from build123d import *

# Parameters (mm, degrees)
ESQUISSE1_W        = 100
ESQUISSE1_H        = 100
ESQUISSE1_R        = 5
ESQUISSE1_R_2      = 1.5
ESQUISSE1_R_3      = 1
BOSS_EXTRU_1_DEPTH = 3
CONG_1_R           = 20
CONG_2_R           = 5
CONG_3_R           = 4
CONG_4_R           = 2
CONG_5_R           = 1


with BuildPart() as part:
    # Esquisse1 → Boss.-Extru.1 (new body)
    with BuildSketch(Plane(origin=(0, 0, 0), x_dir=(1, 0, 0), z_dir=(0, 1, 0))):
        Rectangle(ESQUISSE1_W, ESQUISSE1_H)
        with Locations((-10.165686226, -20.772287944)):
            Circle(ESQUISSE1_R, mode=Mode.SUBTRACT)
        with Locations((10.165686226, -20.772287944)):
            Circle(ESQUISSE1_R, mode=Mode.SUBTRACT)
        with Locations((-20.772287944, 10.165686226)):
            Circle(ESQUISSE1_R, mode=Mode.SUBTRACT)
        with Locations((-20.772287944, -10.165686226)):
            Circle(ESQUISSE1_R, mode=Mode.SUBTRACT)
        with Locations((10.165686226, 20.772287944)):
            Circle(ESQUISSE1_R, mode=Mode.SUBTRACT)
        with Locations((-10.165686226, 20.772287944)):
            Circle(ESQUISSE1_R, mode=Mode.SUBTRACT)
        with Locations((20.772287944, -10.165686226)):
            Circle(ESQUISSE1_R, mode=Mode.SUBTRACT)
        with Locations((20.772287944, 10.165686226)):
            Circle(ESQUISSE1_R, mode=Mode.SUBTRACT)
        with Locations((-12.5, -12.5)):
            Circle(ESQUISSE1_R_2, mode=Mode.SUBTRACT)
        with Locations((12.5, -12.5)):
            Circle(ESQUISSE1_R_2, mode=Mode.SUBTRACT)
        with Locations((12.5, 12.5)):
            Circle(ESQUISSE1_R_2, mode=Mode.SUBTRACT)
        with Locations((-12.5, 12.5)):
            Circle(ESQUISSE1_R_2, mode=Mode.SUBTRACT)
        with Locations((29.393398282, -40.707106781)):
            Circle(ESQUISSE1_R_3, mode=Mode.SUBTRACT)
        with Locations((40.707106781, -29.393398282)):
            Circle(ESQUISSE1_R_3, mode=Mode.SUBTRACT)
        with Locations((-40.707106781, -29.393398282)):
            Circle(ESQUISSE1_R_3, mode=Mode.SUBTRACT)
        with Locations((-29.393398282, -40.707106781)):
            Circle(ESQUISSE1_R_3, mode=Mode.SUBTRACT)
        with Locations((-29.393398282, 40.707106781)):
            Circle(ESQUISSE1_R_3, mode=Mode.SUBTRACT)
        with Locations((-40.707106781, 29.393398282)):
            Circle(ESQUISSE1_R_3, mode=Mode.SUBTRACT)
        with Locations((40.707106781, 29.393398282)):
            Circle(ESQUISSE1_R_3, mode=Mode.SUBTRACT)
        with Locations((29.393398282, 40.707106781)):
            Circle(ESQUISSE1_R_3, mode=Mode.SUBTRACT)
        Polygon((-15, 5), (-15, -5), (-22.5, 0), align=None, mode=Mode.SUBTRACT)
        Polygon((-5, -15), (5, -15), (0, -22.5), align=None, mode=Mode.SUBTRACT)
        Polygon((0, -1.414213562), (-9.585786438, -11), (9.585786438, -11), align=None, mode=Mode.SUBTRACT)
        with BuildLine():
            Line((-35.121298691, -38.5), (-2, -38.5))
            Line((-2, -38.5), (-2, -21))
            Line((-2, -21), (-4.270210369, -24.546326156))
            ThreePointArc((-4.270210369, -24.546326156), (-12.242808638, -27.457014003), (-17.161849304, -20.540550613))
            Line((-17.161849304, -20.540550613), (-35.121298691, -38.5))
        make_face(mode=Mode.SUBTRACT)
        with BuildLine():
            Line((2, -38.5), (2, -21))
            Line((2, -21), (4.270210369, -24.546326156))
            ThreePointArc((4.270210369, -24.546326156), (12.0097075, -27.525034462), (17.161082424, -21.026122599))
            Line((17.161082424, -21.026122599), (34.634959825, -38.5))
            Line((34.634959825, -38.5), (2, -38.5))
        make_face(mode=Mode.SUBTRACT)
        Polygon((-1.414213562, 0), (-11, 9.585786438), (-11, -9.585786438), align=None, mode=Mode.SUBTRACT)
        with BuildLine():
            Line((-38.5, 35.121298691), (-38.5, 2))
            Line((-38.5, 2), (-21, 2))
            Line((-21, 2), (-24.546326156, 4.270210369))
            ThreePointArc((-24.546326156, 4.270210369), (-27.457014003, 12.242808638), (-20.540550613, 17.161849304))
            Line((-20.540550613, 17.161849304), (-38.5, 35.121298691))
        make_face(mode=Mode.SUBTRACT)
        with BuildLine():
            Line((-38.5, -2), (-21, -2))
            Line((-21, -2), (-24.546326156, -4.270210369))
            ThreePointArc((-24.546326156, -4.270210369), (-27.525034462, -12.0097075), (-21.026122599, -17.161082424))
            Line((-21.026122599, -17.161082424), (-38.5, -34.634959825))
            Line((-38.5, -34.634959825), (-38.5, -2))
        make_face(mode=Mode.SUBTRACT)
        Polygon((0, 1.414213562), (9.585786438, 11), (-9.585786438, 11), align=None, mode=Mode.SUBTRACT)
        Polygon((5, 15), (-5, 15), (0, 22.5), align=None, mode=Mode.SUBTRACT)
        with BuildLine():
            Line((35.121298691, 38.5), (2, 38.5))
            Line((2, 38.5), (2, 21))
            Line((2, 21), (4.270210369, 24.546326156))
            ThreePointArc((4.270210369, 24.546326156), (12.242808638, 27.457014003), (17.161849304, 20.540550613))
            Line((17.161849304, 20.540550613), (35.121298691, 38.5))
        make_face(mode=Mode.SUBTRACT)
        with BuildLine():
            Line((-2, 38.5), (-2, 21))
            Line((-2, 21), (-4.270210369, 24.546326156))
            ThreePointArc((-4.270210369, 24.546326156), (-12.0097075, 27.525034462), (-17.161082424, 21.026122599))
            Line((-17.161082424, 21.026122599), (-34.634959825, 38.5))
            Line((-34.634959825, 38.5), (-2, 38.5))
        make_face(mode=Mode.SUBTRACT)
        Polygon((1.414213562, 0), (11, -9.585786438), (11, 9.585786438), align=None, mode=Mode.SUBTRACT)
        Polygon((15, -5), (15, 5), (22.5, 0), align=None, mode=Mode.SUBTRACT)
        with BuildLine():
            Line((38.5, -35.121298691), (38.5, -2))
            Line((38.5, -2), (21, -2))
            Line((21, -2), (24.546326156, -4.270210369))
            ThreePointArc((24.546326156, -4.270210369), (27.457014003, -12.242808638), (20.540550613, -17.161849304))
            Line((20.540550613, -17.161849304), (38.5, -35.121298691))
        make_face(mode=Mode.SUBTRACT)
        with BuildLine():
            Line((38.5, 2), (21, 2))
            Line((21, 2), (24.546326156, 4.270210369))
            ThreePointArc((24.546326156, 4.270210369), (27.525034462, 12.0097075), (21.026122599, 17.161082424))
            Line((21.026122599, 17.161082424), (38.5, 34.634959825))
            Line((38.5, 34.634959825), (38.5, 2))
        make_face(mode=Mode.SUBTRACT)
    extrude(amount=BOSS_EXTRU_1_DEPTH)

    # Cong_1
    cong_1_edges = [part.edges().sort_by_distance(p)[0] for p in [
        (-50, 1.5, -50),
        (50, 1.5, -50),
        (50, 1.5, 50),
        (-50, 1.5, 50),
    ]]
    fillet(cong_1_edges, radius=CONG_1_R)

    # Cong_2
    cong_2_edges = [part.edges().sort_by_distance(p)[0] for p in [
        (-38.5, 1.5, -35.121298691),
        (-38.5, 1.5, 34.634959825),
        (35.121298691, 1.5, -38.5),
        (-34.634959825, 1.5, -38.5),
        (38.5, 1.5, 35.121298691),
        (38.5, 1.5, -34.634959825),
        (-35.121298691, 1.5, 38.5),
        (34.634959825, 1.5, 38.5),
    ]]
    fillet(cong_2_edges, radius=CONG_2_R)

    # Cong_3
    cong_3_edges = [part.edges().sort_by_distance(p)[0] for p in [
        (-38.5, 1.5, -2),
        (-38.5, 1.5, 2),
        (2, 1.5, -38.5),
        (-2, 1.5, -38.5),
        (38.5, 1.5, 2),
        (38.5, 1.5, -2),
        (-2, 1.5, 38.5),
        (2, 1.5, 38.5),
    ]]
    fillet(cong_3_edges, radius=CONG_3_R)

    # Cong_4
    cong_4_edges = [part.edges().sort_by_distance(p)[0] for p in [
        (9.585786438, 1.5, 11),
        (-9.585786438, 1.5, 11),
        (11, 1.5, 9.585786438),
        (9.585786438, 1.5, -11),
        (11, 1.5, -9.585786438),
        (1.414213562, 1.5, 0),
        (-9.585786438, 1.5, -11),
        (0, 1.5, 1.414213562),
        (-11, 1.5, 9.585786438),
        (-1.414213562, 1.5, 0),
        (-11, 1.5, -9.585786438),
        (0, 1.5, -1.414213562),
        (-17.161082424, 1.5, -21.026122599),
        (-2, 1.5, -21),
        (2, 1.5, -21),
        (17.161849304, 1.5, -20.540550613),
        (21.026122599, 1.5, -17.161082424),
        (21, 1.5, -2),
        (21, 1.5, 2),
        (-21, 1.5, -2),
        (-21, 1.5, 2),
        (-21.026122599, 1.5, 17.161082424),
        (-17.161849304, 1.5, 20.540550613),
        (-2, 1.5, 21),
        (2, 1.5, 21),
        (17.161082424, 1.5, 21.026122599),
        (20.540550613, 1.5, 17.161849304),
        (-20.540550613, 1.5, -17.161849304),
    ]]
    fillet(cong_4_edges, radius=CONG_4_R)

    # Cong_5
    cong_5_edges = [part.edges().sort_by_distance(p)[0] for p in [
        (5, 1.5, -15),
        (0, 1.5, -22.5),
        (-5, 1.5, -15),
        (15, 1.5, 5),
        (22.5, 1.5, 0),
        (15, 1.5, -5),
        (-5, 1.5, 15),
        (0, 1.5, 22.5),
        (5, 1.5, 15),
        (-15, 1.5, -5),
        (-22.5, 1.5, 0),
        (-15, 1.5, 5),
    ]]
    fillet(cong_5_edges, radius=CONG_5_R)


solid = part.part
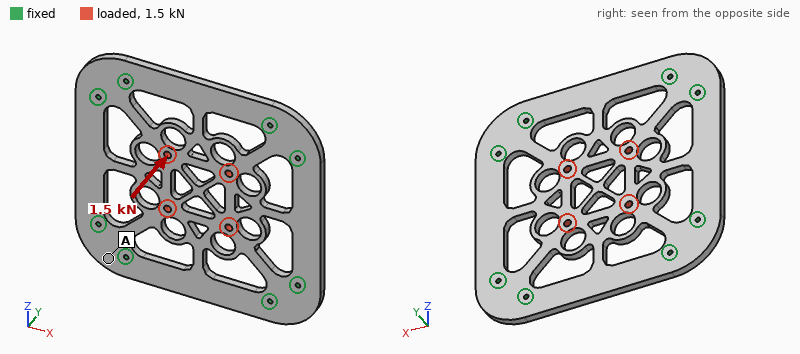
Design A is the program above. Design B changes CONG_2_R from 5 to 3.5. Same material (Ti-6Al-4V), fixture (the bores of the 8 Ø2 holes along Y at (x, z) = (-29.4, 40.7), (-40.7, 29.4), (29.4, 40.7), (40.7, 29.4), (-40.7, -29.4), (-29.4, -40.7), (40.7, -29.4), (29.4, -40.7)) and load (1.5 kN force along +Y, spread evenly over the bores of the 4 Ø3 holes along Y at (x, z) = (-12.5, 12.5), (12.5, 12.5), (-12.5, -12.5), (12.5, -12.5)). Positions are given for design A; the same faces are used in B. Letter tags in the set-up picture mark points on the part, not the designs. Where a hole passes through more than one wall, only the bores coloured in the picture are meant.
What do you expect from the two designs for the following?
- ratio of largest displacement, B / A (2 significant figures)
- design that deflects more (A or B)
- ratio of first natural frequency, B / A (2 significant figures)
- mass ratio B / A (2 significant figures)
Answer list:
1.1
B
0.95
0.98
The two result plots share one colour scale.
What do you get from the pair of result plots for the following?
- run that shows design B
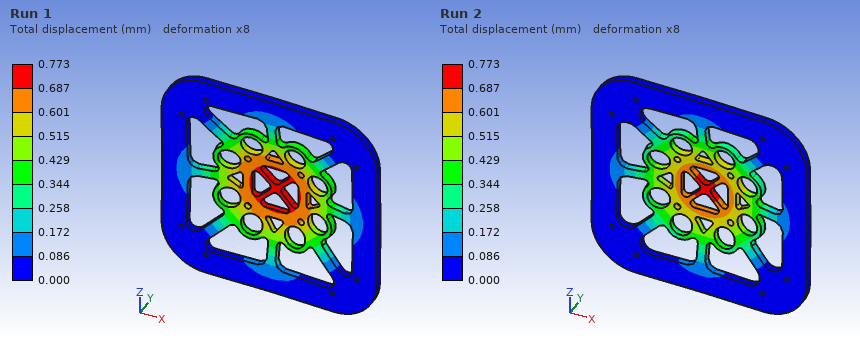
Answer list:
Run 1
